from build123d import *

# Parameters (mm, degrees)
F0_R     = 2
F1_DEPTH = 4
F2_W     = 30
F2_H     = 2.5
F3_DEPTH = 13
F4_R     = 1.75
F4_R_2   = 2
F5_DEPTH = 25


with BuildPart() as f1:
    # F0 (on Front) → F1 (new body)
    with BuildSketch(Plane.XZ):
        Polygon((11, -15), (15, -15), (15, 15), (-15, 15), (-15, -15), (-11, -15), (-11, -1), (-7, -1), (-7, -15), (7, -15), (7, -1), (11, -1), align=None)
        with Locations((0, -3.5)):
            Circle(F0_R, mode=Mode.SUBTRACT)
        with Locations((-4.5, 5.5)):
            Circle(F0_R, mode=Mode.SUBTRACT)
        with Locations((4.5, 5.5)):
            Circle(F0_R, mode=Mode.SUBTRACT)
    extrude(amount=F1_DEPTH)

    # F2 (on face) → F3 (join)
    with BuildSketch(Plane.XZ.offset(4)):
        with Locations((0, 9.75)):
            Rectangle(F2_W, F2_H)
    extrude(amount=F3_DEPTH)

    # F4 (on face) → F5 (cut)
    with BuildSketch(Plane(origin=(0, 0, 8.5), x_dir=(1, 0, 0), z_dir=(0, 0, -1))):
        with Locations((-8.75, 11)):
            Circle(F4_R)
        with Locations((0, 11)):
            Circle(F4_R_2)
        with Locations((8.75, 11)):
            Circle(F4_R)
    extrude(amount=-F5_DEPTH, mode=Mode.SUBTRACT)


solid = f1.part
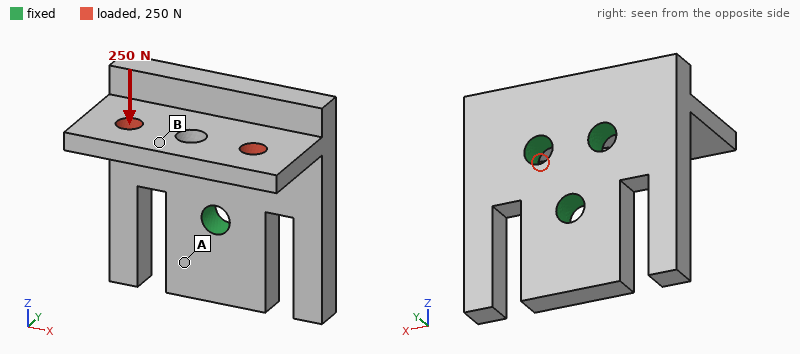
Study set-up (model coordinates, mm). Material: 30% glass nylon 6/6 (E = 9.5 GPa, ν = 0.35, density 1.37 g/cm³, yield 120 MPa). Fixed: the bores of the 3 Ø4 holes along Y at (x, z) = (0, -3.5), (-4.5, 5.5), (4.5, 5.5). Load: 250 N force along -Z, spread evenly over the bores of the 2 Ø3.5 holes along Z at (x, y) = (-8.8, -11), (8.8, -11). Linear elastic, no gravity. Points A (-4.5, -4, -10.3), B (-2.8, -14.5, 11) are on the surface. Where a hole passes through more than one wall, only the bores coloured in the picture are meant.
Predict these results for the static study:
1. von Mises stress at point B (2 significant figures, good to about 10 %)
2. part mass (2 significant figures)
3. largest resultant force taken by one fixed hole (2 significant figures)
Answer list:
8.1 MPa
5.3 g
120 N
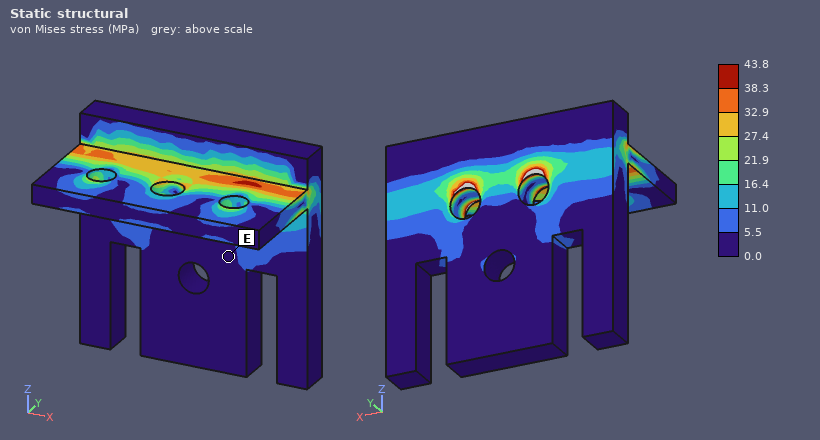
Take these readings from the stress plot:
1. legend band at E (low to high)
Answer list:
0.0 to 5.5 MPa
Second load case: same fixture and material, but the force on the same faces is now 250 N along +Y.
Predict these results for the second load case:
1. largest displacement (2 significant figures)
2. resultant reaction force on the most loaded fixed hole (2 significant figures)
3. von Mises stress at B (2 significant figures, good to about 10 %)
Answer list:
27 µm
130 N
2.6 MPa
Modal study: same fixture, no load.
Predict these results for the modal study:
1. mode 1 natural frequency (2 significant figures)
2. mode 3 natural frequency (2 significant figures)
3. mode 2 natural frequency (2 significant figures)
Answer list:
4400 Hz
5000 Hz
4500 Hz
